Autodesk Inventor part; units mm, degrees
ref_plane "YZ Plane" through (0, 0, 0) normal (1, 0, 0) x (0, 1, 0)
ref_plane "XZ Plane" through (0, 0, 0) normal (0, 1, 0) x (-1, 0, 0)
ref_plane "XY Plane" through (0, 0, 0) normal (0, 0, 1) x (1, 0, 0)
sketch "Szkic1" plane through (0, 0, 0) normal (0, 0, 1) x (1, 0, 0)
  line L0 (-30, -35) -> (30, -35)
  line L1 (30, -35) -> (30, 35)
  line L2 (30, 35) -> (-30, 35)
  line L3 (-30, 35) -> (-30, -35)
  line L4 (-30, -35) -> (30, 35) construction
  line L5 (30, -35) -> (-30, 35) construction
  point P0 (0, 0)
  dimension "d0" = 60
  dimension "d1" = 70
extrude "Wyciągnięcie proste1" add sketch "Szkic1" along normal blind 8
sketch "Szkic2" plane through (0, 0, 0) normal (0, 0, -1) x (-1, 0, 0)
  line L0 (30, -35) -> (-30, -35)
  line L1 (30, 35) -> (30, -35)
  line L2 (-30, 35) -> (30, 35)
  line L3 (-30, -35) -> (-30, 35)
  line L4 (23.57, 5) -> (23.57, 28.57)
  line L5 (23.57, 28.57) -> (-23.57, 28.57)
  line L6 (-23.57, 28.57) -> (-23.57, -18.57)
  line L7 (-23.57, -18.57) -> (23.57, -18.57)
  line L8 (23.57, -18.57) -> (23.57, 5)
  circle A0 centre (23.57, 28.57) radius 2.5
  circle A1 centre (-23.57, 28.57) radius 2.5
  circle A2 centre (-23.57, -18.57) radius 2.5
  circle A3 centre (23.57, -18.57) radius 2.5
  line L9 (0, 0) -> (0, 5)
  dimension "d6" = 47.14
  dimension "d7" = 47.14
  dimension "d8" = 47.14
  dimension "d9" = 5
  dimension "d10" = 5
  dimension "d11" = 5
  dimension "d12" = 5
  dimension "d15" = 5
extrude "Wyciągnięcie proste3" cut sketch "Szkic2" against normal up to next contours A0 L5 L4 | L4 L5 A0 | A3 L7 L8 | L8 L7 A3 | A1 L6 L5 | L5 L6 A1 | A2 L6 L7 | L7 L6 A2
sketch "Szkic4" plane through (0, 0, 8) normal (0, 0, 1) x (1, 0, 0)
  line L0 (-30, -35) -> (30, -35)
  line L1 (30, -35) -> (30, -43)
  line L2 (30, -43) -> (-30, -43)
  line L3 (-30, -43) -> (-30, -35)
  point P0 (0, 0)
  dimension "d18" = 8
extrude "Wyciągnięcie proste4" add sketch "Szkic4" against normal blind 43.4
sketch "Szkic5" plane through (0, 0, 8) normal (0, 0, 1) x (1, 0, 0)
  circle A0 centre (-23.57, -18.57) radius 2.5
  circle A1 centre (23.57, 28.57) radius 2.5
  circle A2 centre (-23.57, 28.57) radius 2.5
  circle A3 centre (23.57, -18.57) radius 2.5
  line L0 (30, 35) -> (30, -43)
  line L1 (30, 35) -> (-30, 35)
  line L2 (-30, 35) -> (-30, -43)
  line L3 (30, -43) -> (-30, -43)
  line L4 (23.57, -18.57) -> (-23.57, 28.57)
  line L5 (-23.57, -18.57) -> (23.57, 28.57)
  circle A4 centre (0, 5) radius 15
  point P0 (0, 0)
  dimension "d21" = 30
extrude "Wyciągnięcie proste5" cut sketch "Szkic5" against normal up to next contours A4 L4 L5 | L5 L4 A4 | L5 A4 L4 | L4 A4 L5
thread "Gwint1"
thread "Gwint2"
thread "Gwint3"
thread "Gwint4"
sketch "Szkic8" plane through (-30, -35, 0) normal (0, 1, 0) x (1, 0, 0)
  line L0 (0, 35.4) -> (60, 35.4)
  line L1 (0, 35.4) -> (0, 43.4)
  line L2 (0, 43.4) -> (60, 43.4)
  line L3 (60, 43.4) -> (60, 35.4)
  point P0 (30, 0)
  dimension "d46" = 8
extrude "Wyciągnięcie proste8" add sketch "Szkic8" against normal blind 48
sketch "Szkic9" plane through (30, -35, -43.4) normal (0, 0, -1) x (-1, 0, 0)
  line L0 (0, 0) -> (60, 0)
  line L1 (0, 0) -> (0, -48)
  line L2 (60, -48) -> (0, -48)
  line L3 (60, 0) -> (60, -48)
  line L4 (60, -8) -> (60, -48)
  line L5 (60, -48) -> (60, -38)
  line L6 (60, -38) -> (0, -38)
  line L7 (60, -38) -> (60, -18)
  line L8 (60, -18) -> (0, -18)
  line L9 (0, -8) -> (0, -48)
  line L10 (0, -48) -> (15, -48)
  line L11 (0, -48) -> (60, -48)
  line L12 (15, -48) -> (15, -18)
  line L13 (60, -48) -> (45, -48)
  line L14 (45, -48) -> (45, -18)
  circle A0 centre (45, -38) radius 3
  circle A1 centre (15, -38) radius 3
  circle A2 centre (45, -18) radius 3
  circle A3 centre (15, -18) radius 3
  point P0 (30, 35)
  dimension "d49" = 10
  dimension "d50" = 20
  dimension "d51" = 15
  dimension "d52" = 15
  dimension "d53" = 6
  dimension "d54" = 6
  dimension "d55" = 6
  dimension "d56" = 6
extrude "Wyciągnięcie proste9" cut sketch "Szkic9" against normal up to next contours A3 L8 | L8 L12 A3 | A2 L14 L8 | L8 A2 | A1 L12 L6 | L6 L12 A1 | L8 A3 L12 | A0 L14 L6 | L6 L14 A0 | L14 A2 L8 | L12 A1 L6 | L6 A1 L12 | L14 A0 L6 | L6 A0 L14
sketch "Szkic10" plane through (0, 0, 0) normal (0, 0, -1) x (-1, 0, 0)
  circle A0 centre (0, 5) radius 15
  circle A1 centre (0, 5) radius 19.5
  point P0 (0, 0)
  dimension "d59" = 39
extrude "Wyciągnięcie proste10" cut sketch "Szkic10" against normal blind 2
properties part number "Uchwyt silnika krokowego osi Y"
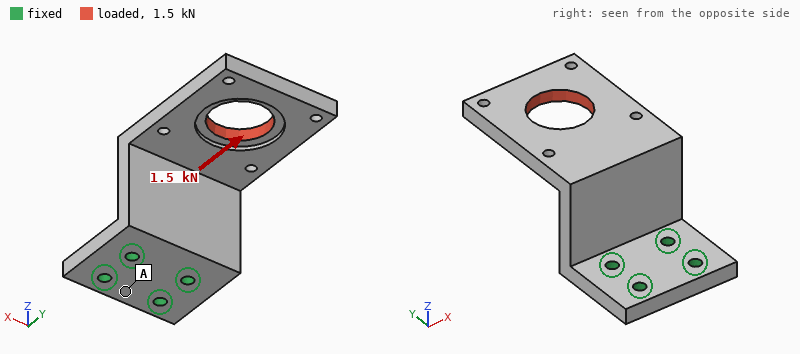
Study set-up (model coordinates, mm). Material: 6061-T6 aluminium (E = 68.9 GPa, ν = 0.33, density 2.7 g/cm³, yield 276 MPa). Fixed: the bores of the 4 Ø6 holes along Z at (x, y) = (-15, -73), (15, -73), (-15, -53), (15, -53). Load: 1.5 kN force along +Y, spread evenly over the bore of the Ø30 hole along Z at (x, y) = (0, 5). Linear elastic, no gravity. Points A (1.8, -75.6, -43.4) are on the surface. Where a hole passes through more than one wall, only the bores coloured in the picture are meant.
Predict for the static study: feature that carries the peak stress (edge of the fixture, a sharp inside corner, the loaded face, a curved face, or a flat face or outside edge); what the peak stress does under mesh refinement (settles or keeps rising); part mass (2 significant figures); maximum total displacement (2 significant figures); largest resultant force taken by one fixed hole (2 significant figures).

edge of the fixture
keeps rising
190 g
1.1 mm
870 N
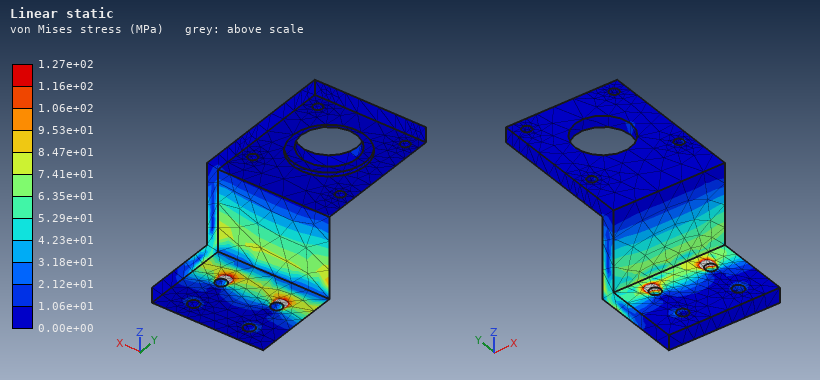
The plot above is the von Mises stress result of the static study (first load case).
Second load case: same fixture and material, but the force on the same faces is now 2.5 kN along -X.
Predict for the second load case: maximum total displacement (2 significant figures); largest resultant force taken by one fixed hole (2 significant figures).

0.94 mm
4.5 kN
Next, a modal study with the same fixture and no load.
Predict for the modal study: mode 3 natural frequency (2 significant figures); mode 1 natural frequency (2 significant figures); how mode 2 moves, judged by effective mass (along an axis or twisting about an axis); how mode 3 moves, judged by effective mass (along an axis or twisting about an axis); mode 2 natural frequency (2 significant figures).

1700 Hz
580 Hz
along X
along Y
1200 Hz
